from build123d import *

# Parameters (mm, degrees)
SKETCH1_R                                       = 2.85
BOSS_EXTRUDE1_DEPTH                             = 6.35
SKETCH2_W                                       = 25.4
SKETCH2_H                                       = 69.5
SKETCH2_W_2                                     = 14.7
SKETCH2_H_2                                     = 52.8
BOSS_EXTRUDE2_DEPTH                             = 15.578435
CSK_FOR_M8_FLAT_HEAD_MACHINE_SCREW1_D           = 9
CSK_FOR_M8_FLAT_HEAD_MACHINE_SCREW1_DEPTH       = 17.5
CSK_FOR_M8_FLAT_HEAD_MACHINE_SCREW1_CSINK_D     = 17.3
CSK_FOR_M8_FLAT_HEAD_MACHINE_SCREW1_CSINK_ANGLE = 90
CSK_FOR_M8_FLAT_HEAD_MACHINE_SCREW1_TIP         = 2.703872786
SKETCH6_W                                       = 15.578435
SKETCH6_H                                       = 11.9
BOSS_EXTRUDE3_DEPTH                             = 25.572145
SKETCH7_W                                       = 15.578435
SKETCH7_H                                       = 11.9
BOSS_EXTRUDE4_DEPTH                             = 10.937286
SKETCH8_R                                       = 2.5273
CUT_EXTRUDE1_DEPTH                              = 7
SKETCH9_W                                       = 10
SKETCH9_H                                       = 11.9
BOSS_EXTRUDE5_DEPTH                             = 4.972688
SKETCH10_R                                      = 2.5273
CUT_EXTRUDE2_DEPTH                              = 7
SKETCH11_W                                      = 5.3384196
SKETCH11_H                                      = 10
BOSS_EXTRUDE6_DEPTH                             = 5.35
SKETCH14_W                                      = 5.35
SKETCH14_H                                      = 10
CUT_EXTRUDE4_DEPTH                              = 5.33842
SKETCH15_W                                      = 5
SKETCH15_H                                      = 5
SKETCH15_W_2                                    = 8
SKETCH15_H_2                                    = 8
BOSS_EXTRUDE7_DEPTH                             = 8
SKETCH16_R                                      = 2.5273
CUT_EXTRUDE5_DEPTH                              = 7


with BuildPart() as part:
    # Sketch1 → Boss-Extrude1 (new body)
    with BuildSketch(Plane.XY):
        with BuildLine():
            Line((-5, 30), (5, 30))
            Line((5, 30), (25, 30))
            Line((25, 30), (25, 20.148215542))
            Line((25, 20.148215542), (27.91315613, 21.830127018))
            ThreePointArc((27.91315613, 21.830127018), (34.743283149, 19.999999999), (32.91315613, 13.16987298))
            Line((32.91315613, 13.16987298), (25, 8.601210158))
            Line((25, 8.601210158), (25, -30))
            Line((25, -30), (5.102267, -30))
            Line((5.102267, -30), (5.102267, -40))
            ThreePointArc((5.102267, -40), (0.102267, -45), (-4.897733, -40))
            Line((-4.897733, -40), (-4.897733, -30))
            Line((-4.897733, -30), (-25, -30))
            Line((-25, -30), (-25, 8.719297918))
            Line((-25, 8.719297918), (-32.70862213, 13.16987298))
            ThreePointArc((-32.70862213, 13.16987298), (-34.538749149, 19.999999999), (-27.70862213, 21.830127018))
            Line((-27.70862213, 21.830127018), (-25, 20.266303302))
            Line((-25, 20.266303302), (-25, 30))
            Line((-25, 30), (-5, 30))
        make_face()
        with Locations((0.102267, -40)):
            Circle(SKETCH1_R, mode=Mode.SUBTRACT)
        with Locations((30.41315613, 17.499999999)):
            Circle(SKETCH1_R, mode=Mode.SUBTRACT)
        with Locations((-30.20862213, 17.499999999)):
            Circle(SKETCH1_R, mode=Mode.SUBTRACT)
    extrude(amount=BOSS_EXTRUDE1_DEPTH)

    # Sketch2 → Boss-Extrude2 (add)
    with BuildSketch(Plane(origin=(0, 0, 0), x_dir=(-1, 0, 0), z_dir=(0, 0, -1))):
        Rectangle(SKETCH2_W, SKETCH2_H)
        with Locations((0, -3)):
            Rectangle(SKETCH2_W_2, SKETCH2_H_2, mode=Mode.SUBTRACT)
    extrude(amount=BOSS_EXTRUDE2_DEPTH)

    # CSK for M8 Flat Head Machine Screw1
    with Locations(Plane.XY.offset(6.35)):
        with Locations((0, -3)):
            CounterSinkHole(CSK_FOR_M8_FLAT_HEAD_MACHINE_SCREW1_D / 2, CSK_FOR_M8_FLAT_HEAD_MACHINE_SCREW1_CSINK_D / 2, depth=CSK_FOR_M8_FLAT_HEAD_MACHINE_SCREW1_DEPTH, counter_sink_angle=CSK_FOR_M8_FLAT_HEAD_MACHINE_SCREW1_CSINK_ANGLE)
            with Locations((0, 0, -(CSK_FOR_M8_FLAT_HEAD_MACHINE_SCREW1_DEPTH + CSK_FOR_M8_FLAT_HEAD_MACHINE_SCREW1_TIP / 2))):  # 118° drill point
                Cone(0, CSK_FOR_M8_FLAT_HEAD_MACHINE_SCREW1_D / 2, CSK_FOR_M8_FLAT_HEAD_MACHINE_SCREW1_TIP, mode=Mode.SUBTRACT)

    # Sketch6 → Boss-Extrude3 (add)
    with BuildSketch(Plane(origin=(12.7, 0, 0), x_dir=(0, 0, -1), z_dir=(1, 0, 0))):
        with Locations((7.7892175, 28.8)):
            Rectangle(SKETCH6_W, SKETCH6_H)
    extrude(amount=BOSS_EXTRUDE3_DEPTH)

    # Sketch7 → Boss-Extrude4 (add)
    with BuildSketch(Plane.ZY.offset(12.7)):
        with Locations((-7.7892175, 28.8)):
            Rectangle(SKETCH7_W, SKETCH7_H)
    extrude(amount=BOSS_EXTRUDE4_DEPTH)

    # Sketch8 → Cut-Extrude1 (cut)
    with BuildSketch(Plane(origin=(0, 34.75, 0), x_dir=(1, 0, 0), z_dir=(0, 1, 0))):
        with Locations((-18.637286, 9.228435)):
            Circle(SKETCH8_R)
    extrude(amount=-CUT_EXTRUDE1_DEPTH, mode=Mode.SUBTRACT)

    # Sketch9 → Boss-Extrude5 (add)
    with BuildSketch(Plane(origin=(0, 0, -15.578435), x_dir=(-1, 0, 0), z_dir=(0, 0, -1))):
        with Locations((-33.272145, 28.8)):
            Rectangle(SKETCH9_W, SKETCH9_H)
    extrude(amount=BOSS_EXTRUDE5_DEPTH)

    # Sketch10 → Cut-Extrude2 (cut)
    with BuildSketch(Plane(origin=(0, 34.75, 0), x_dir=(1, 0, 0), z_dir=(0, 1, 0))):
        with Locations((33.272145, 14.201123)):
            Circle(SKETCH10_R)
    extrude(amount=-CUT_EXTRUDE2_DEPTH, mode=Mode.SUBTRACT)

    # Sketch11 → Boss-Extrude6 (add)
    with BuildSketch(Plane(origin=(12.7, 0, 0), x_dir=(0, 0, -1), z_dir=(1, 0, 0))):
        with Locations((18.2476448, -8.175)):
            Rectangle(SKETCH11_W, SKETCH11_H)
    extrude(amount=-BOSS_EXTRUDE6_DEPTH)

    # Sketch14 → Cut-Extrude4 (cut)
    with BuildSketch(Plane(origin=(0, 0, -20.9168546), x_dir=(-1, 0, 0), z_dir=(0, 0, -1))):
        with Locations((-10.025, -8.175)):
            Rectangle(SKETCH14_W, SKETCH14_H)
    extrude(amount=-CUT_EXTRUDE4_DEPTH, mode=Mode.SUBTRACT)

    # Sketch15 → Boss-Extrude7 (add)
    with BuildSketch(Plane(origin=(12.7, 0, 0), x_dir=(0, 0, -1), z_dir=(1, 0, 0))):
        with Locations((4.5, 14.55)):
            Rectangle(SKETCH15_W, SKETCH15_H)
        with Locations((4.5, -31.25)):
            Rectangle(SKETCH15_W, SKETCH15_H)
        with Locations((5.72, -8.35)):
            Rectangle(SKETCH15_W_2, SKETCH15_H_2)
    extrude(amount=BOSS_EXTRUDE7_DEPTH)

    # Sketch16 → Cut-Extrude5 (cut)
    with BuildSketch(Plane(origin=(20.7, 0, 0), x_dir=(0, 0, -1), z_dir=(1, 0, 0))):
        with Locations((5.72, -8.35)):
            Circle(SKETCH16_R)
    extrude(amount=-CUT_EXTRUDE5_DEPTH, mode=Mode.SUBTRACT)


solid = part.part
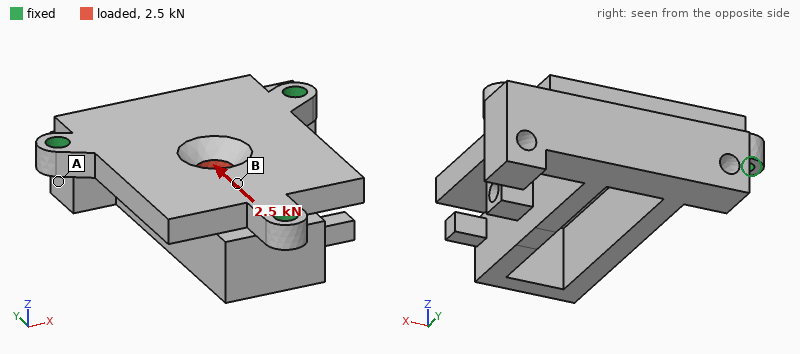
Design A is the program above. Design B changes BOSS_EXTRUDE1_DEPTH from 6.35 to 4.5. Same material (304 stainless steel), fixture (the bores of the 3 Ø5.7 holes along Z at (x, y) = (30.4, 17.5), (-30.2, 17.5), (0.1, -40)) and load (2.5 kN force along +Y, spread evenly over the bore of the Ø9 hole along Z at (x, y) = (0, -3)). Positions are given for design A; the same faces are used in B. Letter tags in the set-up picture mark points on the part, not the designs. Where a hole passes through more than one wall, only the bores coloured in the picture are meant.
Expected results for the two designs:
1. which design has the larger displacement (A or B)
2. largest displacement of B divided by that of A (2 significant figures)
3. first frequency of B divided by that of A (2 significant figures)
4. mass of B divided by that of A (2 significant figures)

B
1.2
0.80
0.87
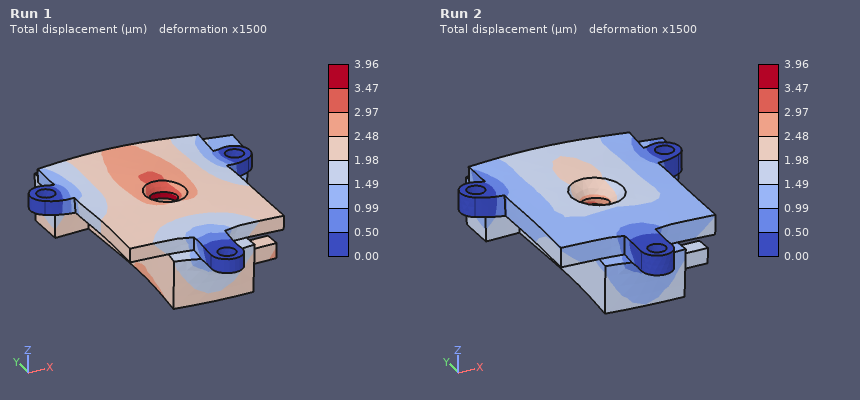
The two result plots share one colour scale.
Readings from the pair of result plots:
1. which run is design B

Run 1
